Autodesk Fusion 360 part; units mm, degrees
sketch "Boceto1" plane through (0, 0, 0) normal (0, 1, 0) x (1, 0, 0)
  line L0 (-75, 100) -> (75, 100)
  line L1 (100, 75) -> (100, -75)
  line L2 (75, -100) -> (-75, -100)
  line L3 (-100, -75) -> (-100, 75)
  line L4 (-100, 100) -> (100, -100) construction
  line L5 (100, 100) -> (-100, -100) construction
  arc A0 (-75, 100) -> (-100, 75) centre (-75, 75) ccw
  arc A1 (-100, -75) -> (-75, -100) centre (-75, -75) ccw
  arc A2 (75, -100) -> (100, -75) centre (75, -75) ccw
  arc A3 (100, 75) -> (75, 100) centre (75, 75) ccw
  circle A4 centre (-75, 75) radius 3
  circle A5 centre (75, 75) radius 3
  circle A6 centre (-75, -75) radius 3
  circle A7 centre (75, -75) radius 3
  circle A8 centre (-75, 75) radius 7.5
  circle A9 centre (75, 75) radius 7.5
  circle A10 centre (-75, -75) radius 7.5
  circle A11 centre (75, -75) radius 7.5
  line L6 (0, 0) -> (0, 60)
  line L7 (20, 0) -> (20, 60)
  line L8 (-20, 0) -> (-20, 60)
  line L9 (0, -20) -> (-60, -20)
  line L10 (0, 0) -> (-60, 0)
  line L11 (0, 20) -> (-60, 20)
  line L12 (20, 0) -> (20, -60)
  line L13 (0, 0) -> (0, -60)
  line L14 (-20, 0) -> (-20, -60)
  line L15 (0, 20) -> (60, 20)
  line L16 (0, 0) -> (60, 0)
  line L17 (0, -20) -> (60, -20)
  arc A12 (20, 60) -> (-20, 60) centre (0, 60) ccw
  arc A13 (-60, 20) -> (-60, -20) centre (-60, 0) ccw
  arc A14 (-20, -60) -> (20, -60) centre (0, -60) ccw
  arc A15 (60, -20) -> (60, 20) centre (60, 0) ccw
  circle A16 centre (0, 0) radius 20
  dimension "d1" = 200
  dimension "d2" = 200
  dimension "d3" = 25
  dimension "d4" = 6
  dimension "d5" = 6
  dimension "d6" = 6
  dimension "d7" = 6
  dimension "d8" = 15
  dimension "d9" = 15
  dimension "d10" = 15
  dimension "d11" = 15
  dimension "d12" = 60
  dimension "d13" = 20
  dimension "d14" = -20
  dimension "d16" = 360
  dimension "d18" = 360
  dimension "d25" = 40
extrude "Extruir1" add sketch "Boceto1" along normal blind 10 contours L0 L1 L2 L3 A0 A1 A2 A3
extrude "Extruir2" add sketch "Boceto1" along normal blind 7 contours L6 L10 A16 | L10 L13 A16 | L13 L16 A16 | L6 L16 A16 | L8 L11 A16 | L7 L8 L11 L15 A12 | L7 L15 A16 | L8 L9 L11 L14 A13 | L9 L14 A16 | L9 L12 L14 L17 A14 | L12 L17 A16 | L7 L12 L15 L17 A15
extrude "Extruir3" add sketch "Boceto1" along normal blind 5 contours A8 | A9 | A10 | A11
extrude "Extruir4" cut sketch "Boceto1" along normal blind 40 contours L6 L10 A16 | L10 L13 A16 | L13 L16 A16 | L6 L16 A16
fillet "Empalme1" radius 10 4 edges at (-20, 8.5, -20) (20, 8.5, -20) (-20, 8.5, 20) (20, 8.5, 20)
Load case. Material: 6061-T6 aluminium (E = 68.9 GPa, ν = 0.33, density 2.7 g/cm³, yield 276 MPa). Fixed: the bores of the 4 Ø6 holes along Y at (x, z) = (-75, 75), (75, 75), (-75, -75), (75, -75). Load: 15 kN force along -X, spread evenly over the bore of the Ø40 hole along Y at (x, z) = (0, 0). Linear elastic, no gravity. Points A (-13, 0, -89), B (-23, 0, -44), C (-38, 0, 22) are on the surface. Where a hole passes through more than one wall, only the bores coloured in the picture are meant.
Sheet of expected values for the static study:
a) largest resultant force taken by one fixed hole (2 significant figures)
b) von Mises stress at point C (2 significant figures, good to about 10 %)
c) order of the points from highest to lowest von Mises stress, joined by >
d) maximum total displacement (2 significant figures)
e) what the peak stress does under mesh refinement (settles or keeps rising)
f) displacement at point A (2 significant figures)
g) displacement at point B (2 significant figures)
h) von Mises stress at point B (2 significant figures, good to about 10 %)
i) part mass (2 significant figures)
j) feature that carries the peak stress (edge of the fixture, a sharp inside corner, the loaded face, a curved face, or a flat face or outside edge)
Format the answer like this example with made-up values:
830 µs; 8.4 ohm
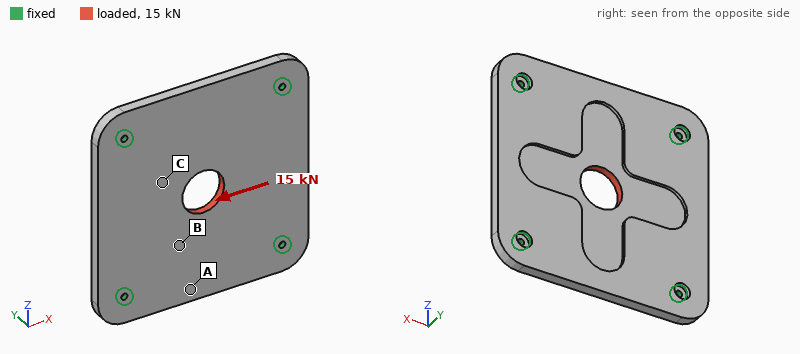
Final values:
3.9 kN; 12 MPa; C > B > A; 24 µm; keeps rising; 8.1 µm; 14 µm; 9.4 MPa; 940 g; edge of the fixture
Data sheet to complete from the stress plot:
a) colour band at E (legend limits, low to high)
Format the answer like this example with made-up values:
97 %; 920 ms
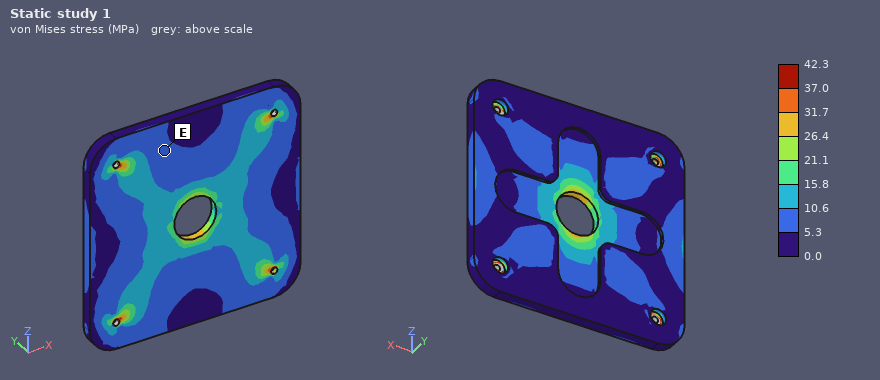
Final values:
5.3 to 10.6 MPa
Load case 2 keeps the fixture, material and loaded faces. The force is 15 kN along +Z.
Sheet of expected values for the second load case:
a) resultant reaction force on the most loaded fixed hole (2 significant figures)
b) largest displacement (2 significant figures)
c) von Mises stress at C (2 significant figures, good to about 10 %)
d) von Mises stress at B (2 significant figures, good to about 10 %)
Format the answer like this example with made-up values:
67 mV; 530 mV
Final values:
3.9 kN; 24 µm; 10 MPa; 11 MPa
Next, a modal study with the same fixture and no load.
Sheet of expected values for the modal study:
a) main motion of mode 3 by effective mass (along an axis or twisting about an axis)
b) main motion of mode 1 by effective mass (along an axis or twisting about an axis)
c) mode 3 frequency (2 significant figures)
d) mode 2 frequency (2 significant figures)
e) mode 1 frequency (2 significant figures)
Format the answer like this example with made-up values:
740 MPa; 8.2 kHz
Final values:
twisting about X; along Y; 1700 Hz; 1500 Hz; 1100 Hz
